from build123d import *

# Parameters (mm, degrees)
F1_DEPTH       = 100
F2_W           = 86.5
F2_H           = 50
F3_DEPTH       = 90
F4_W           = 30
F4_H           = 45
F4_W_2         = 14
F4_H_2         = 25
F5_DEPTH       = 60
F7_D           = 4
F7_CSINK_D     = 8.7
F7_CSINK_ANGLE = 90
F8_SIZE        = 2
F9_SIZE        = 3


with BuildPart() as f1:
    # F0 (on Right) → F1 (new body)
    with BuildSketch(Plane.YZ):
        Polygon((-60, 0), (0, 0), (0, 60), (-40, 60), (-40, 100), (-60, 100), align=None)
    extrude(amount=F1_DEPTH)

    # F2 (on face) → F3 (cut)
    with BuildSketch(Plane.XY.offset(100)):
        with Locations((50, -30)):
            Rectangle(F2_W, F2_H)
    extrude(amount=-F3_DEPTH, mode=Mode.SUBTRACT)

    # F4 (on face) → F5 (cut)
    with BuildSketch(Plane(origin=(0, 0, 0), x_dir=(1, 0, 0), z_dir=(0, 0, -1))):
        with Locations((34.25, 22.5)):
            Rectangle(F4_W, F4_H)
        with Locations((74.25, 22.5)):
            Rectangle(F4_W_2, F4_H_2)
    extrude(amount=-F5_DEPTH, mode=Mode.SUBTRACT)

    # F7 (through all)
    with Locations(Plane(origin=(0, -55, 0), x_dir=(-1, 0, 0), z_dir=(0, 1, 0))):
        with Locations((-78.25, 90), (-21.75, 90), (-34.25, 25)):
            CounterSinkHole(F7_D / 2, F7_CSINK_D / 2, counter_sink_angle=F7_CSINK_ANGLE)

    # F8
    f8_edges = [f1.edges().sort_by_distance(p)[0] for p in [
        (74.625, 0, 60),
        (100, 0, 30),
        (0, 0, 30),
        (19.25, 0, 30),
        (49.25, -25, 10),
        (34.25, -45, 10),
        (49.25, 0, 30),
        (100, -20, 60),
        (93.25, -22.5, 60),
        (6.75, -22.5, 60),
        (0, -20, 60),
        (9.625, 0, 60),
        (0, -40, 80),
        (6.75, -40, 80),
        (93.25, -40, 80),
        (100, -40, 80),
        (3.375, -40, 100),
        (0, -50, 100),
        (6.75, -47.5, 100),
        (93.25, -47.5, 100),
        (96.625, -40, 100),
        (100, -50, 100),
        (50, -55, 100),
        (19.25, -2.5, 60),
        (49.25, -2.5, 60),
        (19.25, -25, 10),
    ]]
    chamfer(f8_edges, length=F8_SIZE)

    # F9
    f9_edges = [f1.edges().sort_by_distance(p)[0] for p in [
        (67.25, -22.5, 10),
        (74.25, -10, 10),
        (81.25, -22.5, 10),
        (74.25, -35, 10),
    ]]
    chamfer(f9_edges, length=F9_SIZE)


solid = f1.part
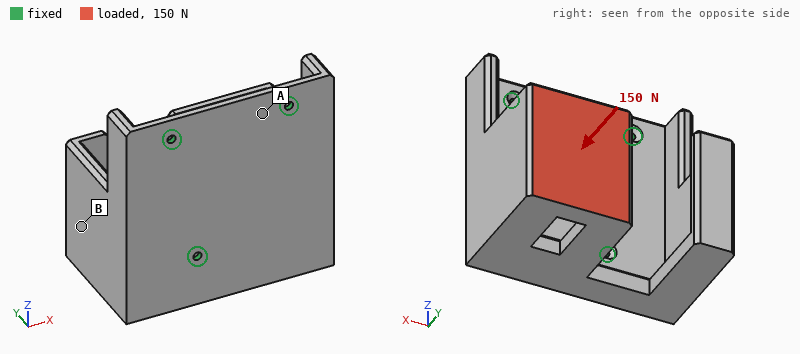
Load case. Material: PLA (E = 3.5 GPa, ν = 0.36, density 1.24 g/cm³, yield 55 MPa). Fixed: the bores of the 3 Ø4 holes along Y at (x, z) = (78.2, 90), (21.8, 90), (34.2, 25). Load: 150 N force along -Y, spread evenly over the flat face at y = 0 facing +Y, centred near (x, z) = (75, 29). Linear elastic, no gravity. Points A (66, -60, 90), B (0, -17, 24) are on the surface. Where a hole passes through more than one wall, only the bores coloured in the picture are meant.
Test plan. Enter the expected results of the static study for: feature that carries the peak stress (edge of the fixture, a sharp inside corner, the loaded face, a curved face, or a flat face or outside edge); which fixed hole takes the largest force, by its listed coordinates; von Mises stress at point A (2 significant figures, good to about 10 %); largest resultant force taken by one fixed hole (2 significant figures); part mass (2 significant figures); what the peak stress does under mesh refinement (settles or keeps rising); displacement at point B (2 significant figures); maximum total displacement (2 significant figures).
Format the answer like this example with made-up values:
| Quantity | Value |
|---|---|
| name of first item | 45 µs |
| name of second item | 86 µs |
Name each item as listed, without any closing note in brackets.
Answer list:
| Quantity | Value |
|---|---|
| feature that carries the peak stress | edge of the fixture |
| which fixed hole takes the largest force, by its listed coordinates | (34.2, 25) |
| von Mises stress at point A | 1.9 MPa |
| largest resultant force taken by one fixed hole | 140 N |
| part mass | 180 g |
| what the peak stress does under mesh refinement | keeps rising |
| displacement at point B | 0.58 mm |
| maximum total displacement | 1.5 mm |
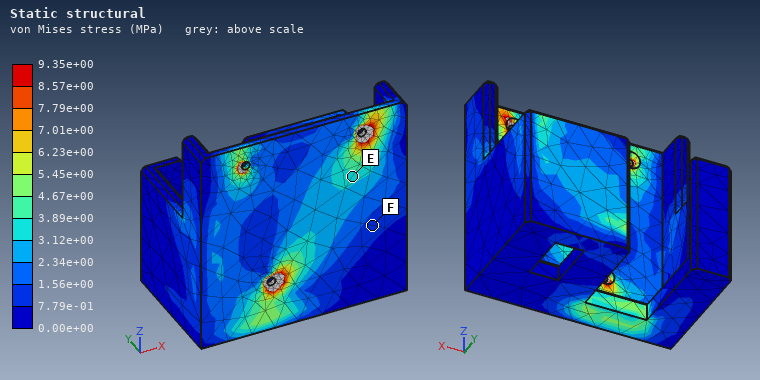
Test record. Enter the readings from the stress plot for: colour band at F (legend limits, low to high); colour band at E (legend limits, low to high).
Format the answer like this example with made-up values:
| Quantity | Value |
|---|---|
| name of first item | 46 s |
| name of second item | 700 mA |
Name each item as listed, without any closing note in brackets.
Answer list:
| Quantity | Value |
|---|---|
| colour band at F | 7.79e-01 to 1.56e+00 MPa |
| colour band at E | 3.12e+00 to 3.89e+00 MPa |
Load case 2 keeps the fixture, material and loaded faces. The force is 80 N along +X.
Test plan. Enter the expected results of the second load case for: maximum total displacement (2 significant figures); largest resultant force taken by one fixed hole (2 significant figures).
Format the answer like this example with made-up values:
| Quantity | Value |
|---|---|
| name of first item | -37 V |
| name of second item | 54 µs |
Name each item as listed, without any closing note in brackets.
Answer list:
| Quantity | Value |
|---|---|
| maximum total displacement | 1.8 mm |
| largest resultant force taken by one fixed hole | 85 N |
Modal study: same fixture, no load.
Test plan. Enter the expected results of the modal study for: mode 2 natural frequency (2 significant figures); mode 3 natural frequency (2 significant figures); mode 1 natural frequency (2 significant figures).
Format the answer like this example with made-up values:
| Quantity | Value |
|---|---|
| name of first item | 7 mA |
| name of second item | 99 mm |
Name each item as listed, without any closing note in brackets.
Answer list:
| Quantity | Value |
|---|---|
| mode 2 natural frequency | 370 Hz |
| mode 3 natural frequency | 440 Hz |
| mode 1 natural frequency | 140 Hz |
